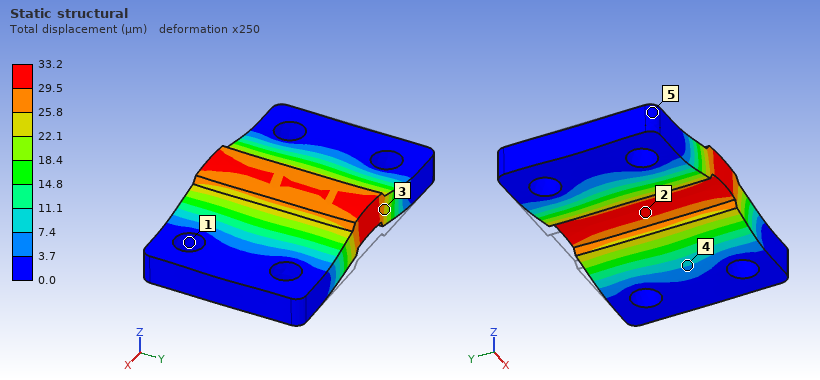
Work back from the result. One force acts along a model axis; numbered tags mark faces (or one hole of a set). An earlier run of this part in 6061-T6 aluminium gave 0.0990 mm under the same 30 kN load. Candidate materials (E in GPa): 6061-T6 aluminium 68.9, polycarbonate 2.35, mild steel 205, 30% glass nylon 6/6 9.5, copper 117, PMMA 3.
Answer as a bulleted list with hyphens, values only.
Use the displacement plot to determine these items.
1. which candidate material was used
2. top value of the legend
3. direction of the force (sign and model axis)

- mild steel
- 33.2 µm
- +Z
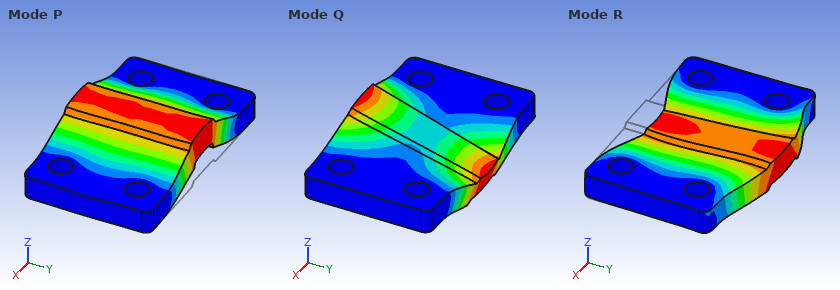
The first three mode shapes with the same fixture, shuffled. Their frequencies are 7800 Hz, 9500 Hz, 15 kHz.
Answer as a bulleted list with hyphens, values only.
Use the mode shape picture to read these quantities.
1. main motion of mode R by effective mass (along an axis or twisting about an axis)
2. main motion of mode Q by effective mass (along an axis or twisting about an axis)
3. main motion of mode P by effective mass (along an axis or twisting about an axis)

- along Y
- twisting about X
- along Z
